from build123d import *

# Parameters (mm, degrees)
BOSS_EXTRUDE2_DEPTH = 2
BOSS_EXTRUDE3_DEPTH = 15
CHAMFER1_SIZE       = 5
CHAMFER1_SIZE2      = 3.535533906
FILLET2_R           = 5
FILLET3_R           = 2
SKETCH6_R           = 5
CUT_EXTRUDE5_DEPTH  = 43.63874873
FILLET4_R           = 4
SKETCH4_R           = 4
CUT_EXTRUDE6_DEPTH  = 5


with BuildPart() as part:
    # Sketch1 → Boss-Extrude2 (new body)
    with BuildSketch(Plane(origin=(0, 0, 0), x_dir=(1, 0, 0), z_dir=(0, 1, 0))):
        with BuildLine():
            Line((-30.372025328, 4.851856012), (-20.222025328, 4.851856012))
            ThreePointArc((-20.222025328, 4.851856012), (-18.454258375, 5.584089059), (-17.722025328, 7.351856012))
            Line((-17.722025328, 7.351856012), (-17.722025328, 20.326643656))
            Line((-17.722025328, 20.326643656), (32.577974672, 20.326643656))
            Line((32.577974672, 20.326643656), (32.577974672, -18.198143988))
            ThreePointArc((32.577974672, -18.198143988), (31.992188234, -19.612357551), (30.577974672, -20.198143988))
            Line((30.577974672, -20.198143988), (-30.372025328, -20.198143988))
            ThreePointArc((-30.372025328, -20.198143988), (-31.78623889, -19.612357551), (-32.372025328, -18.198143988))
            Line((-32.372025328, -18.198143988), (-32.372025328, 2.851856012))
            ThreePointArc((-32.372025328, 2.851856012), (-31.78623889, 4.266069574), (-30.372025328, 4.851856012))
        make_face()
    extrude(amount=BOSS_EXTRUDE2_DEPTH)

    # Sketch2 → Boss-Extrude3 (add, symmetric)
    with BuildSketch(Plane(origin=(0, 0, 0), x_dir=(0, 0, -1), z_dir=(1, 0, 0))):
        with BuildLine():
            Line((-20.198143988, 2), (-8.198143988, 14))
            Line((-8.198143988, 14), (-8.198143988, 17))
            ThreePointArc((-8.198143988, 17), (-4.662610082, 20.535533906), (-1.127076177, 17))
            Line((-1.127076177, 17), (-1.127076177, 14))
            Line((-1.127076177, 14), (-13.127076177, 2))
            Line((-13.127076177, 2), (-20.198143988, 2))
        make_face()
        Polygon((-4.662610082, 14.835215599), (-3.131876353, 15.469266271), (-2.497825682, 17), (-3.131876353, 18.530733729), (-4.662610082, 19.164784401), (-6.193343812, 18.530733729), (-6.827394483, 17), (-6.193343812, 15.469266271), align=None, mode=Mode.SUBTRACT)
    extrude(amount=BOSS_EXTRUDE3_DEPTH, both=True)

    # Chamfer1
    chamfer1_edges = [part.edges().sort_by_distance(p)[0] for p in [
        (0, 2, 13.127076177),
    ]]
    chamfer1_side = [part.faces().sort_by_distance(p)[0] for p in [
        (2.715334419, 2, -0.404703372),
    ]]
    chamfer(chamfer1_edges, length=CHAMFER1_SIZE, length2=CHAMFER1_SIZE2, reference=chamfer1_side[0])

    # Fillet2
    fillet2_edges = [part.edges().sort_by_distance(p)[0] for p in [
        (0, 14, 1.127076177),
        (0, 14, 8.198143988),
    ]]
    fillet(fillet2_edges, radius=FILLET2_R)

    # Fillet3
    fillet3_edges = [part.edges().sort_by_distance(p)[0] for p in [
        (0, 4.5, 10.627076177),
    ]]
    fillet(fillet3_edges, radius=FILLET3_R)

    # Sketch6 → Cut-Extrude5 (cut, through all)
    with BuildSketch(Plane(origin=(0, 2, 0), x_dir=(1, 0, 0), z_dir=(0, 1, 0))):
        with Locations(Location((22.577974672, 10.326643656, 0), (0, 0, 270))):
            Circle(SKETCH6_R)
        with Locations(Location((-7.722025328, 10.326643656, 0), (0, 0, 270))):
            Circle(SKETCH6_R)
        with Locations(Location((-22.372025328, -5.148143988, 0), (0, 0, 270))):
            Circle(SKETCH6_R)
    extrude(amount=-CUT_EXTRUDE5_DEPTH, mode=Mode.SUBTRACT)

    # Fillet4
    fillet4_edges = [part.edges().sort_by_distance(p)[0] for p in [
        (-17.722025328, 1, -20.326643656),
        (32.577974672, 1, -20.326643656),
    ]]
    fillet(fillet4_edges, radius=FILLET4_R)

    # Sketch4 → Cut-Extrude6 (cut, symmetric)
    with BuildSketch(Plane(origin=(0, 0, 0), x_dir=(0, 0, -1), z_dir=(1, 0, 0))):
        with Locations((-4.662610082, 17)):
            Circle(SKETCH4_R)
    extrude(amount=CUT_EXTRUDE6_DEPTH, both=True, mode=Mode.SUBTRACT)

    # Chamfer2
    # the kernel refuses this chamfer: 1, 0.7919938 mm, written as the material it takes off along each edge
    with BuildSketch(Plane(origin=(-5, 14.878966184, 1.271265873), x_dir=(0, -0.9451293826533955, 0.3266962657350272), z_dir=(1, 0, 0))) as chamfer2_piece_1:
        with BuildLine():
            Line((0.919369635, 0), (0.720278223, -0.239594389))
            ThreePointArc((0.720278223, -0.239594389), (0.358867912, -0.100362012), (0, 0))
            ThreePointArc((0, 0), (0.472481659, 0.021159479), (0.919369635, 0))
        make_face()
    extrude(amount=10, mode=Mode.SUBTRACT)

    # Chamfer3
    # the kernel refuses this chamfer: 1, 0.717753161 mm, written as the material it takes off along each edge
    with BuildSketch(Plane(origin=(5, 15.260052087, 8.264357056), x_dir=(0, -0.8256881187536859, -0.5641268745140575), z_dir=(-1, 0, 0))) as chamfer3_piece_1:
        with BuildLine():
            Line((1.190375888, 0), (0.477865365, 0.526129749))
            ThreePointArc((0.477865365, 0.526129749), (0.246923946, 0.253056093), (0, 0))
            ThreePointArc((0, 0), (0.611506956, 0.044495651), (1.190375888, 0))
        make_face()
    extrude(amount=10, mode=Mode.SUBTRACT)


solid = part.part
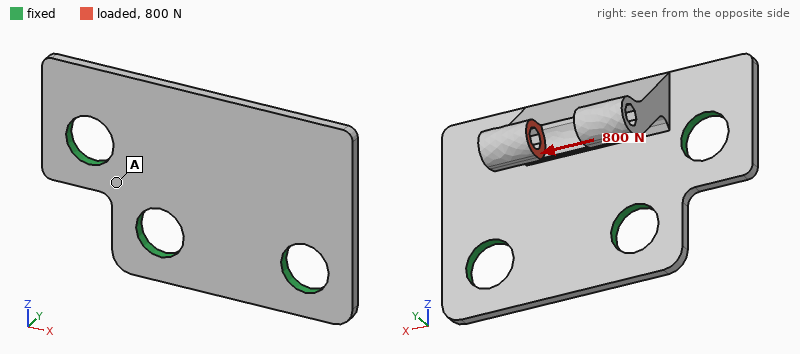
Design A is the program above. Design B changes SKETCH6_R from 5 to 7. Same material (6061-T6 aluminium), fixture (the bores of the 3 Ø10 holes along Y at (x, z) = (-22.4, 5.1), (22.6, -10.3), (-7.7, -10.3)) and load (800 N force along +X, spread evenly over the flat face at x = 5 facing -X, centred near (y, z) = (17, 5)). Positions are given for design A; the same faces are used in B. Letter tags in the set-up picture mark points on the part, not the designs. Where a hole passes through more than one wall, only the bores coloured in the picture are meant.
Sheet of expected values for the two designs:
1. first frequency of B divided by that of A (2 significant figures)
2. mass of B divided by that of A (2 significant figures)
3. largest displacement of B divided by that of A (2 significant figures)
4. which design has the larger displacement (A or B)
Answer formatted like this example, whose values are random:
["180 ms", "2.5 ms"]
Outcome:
["1.2", "0.94", "0.74", "A"]
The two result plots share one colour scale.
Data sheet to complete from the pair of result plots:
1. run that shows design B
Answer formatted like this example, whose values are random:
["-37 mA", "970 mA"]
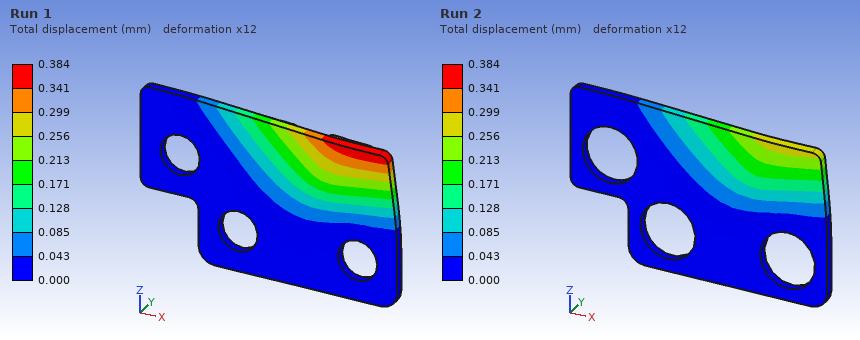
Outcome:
["Run 2"]
